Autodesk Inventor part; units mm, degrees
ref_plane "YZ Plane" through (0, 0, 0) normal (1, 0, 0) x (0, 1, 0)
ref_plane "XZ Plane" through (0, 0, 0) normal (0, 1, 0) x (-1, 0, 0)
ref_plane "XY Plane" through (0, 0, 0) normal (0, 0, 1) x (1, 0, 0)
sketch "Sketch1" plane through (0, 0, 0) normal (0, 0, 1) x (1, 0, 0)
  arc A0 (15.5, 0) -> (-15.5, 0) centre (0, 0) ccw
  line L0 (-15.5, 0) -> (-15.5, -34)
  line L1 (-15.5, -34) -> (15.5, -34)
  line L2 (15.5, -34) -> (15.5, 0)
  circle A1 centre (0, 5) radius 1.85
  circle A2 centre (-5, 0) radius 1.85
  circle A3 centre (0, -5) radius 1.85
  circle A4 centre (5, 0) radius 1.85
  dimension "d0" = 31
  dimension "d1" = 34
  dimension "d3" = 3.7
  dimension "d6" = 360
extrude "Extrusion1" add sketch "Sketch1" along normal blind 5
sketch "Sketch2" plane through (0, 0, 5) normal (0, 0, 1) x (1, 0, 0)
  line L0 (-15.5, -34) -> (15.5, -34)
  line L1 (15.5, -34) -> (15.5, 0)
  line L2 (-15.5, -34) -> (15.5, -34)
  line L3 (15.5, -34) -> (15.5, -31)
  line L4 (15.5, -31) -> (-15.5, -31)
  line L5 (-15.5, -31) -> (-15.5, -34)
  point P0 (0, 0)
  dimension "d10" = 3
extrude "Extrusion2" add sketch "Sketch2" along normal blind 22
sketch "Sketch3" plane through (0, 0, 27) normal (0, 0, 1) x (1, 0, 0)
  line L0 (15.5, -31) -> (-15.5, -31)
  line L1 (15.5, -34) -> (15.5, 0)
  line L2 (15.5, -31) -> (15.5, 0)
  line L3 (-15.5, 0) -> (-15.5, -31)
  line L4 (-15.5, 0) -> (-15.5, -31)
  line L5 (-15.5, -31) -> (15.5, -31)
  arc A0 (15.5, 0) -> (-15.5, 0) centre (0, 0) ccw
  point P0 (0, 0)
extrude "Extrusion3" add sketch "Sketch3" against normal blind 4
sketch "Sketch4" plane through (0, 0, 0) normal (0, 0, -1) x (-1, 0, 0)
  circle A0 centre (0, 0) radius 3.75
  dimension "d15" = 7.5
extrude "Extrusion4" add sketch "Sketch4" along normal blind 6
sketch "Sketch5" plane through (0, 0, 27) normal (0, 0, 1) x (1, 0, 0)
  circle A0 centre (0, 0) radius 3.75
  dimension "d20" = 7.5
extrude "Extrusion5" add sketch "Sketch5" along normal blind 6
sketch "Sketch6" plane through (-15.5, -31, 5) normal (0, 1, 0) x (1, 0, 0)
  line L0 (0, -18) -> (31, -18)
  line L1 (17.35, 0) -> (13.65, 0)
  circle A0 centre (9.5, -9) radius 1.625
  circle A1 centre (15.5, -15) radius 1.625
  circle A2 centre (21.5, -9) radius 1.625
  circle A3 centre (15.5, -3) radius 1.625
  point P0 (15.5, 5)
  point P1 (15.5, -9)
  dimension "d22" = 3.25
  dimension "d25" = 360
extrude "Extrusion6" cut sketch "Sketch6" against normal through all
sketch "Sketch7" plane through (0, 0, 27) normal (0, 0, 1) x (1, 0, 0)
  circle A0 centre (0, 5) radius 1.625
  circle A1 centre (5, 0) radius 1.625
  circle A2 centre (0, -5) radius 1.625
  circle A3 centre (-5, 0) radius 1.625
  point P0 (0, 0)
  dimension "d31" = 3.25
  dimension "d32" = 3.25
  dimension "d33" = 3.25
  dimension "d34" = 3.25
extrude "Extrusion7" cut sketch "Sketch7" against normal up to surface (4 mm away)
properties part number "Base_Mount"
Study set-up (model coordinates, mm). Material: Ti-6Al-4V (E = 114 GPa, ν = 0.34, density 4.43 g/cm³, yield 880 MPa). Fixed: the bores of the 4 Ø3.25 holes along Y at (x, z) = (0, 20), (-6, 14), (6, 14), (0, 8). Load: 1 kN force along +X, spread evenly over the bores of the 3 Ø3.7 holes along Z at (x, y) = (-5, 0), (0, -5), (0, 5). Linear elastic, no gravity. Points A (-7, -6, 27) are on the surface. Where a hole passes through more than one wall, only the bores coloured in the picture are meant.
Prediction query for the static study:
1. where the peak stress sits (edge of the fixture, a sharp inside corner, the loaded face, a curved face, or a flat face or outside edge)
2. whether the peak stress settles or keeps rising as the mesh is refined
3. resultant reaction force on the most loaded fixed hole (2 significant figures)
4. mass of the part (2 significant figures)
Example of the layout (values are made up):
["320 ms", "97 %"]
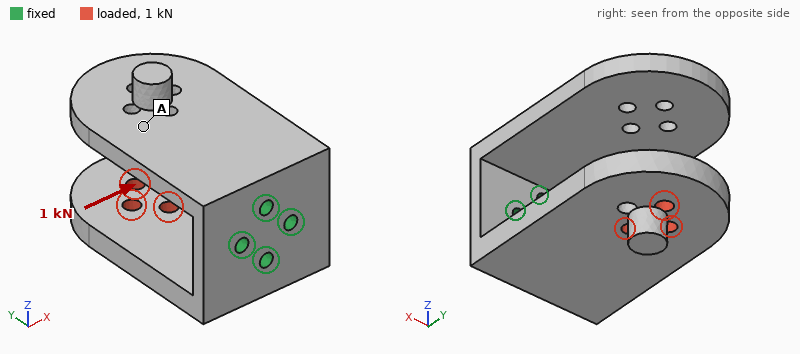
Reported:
["edge of the fixture", "keeps rising", "1.3 kN", "65 g"]
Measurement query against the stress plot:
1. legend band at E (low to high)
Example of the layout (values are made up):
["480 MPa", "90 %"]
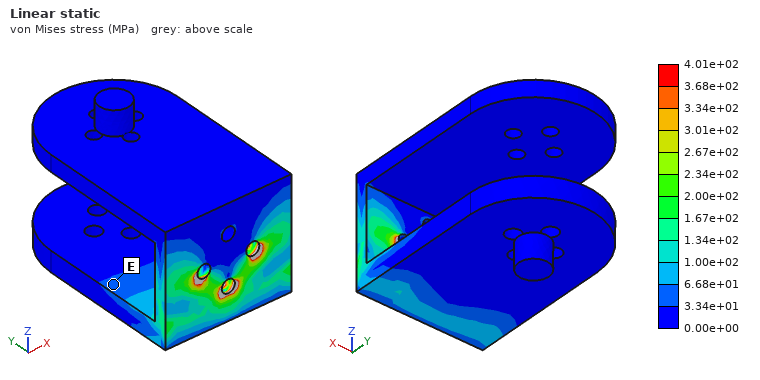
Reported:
["3.34e+01 to 6.68e+01 MPa"]
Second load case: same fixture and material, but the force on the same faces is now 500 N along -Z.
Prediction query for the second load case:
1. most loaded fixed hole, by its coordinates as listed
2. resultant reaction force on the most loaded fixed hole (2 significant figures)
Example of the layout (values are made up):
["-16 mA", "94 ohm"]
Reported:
["(0, 8)", "1.4 kN"]
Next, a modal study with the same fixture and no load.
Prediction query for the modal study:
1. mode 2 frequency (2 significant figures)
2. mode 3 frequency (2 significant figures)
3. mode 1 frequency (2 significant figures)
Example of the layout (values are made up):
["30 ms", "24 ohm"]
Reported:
["1200 Hz", "2100 Hz", "1200 Hz"]
